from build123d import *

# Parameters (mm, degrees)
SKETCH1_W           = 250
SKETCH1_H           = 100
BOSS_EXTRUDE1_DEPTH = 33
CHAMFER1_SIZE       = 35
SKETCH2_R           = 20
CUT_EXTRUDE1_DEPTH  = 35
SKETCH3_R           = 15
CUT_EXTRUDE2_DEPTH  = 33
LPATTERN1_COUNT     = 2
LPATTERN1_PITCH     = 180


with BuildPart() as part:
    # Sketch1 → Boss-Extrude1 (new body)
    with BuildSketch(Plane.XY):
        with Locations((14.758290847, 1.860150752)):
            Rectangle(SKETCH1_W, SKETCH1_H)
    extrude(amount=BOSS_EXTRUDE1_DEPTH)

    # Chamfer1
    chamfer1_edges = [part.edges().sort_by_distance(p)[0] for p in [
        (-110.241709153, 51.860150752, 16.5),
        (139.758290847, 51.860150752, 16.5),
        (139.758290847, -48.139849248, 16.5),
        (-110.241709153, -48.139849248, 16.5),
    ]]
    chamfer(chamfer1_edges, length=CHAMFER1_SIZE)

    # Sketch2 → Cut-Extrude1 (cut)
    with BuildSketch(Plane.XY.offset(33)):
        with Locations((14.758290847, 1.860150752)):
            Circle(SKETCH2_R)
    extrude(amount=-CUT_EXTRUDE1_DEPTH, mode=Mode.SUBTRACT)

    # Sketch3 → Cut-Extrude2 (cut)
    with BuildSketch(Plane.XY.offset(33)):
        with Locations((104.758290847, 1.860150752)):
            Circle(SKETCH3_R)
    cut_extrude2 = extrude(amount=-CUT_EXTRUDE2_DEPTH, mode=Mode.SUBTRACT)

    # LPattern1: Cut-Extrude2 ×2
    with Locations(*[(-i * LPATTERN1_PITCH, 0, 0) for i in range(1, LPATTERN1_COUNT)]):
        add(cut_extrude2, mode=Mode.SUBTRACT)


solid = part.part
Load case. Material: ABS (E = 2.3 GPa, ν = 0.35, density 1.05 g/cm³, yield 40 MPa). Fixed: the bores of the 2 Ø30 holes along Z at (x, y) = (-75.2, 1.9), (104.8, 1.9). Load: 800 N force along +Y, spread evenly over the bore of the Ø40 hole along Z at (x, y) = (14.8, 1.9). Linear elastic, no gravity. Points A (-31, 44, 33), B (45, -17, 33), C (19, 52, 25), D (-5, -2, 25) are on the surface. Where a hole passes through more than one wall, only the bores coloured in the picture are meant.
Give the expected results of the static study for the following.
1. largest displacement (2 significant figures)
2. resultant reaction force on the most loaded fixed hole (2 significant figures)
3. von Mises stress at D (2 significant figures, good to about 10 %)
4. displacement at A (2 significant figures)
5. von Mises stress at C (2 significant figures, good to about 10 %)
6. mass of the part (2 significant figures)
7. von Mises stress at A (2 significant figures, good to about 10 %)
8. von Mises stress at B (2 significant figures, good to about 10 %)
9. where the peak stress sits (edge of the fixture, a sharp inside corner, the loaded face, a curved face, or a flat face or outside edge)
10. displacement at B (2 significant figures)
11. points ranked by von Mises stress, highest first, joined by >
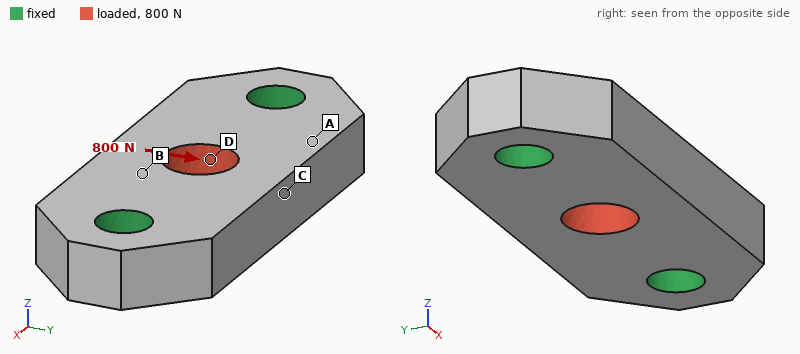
20 µm
400 N
0.35 MPa
11 µm
0.49 MPa
690 g
0.16 MPa
0.27 MPa
edge of the fixture
15 µm
C > D > B > A
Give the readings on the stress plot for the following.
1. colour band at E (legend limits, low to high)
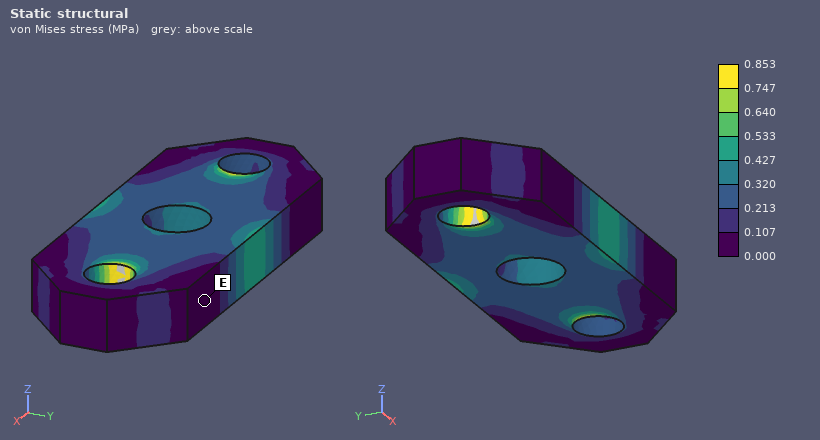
0.000 to 0.107 MPa
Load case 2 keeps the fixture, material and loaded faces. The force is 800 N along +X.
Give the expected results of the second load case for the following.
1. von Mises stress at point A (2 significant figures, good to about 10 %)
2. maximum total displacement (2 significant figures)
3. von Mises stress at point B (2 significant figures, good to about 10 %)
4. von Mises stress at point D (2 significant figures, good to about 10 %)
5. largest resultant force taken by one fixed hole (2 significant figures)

0.054 MPa
6.3 µm
0.19 MPa
0.21 MPa
400 N
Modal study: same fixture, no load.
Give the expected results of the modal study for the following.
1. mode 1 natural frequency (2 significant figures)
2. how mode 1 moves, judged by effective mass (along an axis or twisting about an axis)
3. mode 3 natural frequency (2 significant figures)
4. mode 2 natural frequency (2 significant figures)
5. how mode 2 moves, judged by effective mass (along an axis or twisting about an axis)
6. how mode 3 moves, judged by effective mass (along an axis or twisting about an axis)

1400 Hz
along Z
2100 Hz
1500 Hz
twisting about X
along Y
